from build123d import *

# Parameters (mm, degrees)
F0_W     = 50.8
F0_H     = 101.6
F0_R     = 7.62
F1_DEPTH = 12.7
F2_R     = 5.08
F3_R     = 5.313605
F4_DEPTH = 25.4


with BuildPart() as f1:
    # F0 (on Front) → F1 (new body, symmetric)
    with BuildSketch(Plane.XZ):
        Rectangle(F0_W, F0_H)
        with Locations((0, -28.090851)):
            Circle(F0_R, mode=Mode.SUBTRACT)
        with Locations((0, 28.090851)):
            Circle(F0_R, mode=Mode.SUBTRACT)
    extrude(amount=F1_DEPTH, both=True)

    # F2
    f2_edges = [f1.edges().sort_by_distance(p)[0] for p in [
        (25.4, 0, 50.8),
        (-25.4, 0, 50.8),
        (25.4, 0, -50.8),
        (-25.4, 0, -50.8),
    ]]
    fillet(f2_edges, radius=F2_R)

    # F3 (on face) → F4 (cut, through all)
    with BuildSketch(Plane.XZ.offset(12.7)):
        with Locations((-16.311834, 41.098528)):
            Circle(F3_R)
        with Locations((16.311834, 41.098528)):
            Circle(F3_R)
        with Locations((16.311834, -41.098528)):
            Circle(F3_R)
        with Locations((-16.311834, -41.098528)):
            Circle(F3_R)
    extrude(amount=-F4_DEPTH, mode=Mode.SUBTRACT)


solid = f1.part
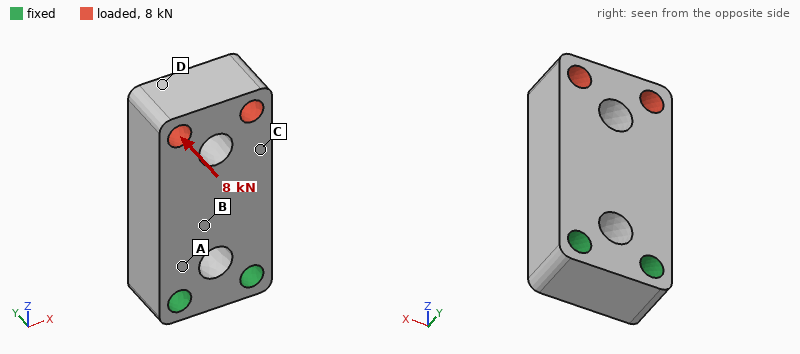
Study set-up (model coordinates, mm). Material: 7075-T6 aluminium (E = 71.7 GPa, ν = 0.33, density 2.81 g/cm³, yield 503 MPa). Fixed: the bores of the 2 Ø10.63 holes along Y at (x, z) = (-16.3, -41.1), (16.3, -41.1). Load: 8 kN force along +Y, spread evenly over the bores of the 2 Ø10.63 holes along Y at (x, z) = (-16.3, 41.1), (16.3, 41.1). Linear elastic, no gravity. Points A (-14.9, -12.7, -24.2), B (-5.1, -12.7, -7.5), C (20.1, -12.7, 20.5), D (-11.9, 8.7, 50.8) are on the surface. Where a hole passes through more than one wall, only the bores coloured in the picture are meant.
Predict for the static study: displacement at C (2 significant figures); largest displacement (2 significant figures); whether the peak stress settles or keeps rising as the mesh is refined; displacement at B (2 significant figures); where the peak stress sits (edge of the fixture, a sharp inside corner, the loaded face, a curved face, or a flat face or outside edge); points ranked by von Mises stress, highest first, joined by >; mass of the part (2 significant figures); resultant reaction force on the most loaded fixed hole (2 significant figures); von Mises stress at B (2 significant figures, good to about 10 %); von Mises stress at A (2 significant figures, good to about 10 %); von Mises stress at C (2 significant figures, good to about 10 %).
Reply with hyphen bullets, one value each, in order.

- 0.23 mm
- 0.42 mm
- keeps rising
- 0.096 mm
- edge of the fixture
- A > B > C > D
- 320 g
- 4.0 kN
- 60 MPa
- 120 MPa
- 37 MPa
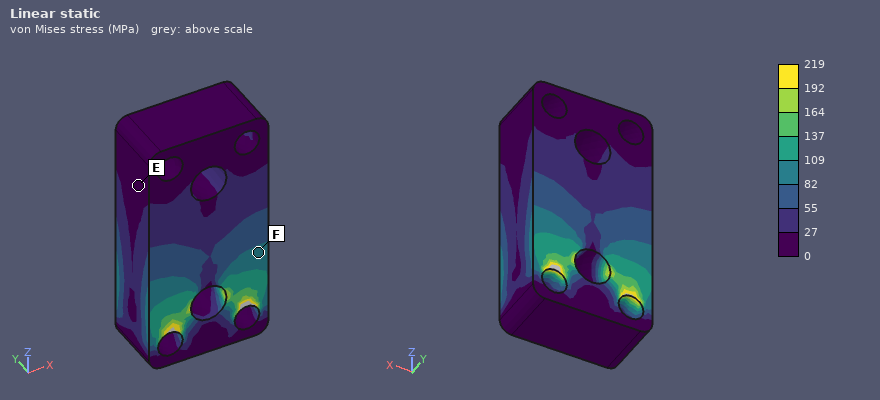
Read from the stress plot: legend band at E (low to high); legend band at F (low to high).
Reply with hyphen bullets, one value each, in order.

- 0 to 27 MPa
- 82 to 109 MPa
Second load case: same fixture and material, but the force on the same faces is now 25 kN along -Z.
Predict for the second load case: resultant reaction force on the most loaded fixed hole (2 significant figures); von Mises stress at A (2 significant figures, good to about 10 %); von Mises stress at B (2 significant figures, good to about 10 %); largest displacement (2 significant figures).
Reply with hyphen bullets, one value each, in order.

- 13 kN
- 23 MPa
- 14 MPa
- 35 µm
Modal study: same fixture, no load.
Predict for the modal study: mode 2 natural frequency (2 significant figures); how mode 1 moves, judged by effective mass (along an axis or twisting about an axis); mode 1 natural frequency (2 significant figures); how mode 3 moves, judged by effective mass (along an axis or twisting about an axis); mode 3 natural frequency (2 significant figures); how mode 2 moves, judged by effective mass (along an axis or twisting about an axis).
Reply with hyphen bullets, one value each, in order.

- 4400 Hz
- along Y
- 2500 Hz
- twisting about Z
- 6800 Hz
- along X
